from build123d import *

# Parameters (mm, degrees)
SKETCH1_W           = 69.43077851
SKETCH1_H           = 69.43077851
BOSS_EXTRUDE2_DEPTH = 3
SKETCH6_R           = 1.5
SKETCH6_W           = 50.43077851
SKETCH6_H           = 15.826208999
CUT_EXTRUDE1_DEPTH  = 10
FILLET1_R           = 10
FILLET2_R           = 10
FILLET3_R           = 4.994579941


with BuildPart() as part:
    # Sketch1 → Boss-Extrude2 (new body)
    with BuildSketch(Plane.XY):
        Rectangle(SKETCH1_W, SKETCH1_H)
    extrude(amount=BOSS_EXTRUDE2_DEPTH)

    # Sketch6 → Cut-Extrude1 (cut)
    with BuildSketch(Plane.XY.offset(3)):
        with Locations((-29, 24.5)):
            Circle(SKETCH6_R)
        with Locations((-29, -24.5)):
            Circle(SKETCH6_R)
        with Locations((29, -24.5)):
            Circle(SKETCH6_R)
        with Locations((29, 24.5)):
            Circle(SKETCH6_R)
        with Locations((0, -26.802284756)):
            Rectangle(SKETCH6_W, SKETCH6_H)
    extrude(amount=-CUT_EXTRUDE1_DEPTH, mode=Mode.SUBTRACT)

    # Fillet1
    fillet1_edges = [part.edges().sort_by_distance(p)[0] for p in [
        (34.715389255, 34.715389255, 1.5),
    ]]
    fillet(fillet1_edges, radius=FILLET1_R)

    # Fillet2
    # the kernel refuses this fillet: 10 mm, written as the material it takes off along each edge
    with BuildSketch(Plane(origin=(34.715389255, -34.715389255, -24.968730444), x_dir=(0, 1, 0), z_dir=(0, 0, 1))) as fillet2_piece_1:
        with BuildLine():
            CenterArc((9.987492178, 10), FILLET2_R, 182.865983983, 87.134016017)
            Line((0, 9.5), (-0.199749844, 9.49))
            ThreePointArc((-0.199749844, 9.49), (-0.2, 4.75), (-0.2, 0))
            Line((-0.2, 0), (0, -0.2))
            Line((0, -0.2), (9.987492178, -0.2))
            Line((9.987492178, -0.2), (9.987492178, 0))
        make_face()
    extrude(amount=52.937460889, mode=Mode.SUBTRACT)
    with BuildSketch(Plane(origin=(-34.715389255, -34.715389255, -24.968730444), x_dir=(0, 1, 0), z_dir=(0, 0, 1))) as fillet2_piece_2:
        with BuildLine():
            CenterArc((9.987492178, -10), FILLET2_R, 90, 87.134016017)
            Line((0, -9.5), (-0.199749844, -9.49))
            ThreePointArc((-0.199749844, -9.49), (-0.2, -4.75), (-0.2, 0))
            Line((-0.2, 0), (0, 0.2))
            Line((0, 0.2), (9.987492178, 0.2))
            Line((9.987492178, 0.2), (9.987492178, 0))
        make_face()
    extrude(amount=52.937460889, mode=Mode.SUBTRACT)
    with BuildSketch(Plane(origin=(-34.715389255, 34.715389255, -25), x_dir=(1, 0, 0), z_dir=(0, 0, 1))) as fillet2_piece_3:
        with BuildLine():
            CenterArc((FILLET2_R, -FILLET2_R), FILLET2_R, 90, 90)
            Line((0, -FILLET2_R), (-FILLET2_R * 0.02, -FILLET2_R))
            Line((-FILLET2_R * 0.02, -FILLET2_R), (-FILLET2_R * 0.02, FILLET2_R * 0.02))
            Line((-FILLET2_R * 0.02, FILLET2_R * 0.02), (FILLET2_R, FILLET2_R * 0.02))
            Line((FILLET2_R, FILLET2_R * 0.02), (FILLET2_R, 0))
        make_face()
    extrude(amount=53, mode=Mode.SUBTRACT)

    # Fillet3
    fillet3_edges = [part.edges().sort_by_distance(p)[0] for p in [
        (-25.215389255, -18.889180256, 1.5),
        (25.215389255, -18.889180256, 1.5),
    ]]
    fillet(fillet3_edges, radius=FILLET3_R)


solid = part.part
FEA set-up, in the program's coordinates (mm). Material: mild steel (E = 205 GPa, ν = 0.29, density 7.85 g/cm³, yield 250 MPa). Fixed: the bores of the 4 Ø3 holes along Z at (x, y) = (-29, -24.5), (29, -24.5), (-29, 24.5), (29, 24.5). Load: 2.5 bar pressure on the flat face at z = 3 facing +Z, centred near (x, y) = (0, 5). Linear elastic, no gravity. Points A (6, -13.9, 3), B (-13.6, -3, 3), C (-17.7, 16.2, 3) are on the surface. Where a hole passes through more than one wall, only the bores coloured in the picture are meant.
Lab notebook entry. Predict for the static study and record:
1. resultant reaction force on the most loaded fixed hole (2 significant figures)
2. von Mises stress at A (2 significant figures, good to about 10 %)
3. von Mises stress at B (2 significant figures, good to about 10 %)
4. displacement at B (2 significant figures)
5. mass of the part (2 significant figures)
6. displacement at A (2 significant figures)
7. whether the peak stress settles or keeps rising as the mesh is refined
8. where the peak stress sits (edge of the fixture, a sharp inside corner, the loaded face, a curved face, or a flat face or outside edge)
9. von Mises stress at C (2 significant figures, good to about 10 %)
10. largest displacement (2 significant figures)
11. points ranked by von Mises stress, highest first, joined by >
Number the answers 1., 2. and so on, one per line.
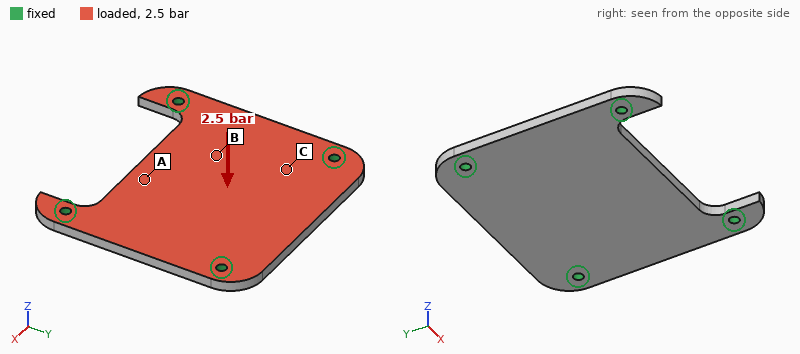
1. 300 N
2. 30 MPa
3. 21 MPa
4. 29 µm
5. 92 g
6. 33 µm
7. keeps rising
8. edge of the fixture
9. 8.7 MPa
10. 36 µm
11. A > B > C
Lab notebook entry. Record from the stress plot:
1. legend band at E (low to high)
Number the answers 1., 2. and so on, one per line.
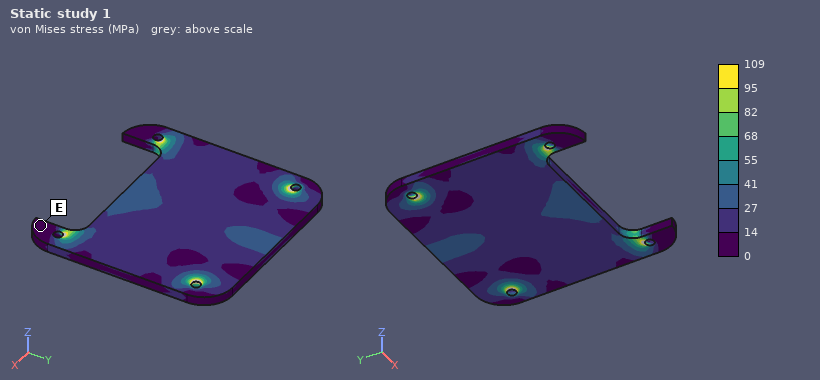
1. 0 to 14 MPa
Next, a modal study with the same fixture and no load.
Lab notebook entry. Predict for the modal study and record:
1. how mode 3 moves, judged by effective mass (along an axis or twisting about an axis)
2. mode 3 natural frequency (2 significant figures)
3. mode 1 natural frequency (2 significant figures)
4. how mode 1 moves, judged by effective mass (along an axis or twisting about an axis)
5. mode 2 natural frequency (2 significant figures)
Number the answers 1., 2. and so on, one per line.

1. twisting about Y
2. 6400 Hz
3. 3200 Hz
4. along Z
5. 5100 Hz
